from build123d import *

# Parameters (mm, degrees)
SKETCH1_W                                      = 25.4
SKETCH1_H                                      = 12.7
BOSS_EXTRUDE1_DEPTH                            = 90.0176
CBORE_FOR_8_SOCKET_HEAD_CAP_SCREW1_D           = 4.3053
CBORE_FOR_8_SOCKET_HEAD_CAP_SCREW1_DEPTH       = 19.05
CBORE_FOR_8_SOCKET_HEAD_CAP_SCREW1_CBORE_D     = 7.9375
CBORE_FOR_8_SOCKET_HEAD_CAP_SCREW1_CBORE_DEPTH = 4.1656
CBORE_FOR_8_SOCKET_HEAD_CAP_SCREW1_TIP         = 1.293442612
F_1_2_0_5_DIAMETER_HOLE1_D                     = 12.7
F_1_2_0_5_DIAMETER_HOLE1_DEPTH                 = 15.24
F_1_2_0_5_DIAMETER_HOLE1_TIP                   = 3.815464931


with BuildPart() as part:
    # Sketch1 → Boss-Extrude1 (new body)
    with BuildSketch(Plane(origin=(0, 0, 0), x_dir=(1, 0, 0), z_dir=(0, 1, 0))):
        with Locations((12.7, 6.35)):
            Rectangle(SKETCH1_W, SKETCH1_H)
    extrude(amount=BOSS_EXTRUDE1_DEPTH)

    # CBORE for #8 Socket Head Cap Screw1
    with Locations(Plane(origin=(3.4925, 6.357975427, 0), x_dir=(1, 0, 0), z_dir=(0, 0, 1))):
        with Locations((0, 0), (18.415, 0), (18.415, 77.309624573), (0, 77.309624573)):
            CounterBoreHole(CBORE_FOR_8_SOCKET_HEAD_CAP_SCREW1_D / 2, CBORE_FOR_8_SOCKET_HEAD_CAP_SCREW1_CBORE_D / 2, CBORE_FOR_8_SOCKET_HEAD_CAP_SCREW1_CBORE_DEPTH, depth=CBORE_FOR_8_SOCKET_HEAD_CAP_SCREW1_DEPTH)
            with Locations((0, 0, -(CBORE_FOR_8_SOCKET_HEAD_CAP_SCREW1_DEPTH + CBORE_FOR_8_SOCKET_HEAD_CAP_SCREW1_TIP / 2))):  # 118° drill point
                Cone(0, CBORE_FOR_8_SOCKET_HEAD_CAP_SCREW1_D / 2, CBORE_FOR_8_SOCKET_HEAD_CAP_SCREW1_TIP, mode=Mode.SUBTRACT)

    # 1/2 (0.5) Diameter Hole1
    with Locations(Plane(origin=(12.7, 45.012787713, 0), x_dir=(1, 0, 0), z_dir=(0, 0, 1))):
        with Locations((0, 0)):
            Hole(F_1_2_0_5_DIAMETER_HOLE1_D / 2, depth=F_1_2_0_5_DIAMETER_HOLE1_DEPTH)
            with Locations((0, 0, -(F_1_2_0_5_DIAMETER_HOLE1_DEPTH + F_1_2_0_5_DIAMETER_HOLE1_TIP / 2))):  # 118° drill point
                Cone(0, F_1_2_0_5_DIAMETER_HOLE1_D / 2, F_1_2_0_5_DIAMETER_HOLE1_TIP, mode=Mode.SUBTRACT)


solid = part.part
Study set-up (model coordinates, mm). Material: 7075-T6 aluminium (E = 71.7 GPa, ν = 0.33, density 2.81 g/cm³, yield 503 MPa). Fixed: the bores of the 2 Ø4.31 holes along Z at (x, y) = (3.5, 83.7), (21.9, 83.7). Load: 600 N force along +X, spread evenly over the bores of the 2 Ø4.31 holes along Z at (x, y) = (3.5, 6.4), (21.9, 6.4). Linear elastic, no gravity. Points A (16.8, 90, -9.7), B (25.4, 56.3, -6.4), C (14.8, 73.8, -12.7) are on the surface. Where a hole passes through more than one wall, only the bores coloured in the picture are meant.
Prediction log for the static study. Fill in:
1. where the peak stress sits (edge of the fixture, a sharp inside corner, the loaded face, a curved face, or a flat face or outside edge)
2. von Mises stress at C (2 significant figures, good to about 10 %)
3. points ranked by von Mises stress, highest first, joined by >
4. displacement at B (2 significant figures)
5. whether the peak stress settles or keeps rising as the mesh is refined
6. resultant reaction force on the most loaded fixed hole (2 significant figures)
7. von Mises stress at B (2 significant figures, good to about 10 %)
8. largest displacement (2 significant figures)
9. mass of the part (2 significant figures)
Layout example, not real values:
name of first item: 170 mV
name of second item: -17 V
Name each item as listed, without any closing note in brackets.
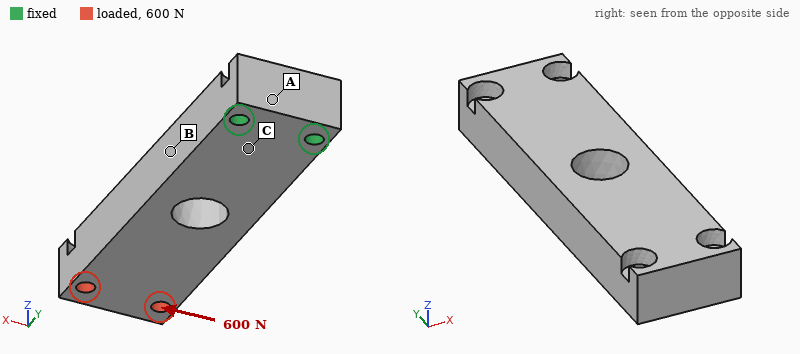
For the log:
where the peak stress sits: edge of the fixture
von Mises stress at C: 13 MPa
points ranked by von Mises stress, highest first, joined by >: B > C > A
displacement at B: 0.021 mm
whether the peak stress settles or keeps rising as the mesh is refined: keeps rising
resultant reaction force on the most loaded fixed hole: 2.4 kN
von Mises stress at B: 26 MPa
largest displacement: 0.11 mm
mass of the part: 73 g
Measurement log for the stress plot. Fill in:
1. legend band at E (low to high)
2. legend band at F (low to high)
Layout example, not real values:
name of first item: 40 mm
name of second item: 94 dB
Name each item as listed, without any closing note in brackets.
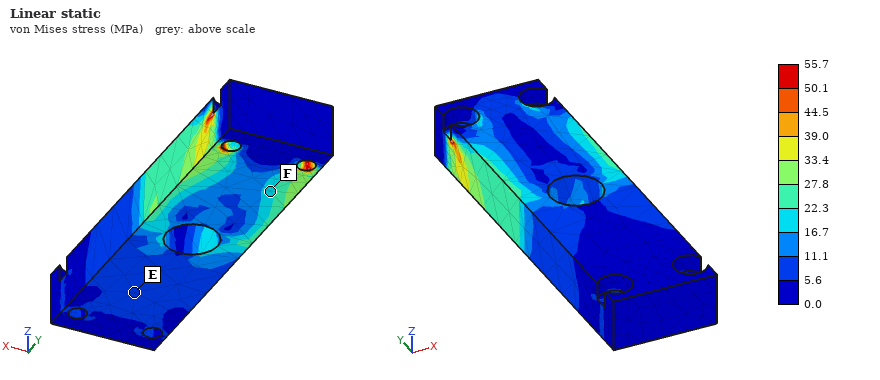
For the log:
legend band at E: 5.6 to 11.1 MPa
legend band at F: 16.7 to 22.3 MPa
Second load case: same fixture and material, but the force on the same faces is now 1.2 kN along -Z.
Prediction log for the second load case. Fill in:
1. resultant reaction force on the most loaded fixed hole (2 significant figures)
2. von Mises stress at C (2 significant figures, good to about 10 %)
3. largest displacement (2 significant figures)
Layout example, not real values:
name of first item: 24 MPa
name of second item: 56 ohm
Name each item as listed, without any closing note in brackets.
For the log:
resultant reaction force on the most loaded fixed hole: 760 N
von Mises stress at C: 120 MPa
largest displacement: 1.0 mm
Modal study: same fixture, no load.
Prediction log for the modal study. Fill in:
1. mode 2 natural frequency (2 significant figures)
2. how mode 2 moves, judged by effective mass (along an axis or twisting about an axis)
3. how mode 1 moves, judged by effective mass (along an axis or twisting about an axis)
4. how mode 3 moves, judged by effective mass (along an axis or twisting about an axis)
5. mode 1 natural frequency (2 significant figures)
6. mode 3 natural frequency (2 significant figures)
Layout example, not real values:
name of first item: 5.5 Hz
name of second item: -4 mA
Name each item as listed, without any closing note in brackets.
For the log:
mode 2 natural frequency: 2700 Hz
how mode 2 moves, judged by effective mass: along X
how mode 1 moves, judged by effective mass: along Z
how mode 3 moves, judged by effective mass: twisting about Y
mode 1 natural frequency: 1200 Hz
mode 3 natural frequency: 6600 Hz
